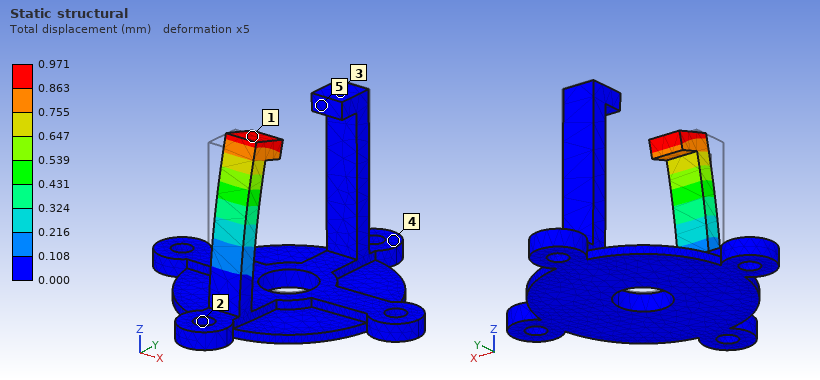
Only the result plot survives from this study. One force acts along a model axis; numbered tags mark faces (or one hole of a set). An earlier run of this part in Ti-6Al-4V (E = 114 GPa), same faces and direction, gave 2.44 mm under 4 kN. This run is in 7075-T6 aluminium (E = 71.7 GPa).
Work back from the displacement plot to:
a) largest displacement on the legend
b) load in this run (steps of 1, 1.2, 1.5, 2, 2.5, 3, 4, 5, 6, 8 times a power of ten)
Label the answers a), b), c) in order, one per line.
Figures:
a) 0.971 mm
b) 1 kN
